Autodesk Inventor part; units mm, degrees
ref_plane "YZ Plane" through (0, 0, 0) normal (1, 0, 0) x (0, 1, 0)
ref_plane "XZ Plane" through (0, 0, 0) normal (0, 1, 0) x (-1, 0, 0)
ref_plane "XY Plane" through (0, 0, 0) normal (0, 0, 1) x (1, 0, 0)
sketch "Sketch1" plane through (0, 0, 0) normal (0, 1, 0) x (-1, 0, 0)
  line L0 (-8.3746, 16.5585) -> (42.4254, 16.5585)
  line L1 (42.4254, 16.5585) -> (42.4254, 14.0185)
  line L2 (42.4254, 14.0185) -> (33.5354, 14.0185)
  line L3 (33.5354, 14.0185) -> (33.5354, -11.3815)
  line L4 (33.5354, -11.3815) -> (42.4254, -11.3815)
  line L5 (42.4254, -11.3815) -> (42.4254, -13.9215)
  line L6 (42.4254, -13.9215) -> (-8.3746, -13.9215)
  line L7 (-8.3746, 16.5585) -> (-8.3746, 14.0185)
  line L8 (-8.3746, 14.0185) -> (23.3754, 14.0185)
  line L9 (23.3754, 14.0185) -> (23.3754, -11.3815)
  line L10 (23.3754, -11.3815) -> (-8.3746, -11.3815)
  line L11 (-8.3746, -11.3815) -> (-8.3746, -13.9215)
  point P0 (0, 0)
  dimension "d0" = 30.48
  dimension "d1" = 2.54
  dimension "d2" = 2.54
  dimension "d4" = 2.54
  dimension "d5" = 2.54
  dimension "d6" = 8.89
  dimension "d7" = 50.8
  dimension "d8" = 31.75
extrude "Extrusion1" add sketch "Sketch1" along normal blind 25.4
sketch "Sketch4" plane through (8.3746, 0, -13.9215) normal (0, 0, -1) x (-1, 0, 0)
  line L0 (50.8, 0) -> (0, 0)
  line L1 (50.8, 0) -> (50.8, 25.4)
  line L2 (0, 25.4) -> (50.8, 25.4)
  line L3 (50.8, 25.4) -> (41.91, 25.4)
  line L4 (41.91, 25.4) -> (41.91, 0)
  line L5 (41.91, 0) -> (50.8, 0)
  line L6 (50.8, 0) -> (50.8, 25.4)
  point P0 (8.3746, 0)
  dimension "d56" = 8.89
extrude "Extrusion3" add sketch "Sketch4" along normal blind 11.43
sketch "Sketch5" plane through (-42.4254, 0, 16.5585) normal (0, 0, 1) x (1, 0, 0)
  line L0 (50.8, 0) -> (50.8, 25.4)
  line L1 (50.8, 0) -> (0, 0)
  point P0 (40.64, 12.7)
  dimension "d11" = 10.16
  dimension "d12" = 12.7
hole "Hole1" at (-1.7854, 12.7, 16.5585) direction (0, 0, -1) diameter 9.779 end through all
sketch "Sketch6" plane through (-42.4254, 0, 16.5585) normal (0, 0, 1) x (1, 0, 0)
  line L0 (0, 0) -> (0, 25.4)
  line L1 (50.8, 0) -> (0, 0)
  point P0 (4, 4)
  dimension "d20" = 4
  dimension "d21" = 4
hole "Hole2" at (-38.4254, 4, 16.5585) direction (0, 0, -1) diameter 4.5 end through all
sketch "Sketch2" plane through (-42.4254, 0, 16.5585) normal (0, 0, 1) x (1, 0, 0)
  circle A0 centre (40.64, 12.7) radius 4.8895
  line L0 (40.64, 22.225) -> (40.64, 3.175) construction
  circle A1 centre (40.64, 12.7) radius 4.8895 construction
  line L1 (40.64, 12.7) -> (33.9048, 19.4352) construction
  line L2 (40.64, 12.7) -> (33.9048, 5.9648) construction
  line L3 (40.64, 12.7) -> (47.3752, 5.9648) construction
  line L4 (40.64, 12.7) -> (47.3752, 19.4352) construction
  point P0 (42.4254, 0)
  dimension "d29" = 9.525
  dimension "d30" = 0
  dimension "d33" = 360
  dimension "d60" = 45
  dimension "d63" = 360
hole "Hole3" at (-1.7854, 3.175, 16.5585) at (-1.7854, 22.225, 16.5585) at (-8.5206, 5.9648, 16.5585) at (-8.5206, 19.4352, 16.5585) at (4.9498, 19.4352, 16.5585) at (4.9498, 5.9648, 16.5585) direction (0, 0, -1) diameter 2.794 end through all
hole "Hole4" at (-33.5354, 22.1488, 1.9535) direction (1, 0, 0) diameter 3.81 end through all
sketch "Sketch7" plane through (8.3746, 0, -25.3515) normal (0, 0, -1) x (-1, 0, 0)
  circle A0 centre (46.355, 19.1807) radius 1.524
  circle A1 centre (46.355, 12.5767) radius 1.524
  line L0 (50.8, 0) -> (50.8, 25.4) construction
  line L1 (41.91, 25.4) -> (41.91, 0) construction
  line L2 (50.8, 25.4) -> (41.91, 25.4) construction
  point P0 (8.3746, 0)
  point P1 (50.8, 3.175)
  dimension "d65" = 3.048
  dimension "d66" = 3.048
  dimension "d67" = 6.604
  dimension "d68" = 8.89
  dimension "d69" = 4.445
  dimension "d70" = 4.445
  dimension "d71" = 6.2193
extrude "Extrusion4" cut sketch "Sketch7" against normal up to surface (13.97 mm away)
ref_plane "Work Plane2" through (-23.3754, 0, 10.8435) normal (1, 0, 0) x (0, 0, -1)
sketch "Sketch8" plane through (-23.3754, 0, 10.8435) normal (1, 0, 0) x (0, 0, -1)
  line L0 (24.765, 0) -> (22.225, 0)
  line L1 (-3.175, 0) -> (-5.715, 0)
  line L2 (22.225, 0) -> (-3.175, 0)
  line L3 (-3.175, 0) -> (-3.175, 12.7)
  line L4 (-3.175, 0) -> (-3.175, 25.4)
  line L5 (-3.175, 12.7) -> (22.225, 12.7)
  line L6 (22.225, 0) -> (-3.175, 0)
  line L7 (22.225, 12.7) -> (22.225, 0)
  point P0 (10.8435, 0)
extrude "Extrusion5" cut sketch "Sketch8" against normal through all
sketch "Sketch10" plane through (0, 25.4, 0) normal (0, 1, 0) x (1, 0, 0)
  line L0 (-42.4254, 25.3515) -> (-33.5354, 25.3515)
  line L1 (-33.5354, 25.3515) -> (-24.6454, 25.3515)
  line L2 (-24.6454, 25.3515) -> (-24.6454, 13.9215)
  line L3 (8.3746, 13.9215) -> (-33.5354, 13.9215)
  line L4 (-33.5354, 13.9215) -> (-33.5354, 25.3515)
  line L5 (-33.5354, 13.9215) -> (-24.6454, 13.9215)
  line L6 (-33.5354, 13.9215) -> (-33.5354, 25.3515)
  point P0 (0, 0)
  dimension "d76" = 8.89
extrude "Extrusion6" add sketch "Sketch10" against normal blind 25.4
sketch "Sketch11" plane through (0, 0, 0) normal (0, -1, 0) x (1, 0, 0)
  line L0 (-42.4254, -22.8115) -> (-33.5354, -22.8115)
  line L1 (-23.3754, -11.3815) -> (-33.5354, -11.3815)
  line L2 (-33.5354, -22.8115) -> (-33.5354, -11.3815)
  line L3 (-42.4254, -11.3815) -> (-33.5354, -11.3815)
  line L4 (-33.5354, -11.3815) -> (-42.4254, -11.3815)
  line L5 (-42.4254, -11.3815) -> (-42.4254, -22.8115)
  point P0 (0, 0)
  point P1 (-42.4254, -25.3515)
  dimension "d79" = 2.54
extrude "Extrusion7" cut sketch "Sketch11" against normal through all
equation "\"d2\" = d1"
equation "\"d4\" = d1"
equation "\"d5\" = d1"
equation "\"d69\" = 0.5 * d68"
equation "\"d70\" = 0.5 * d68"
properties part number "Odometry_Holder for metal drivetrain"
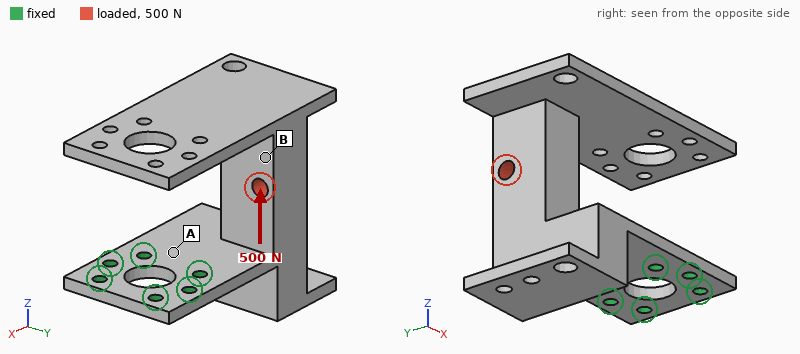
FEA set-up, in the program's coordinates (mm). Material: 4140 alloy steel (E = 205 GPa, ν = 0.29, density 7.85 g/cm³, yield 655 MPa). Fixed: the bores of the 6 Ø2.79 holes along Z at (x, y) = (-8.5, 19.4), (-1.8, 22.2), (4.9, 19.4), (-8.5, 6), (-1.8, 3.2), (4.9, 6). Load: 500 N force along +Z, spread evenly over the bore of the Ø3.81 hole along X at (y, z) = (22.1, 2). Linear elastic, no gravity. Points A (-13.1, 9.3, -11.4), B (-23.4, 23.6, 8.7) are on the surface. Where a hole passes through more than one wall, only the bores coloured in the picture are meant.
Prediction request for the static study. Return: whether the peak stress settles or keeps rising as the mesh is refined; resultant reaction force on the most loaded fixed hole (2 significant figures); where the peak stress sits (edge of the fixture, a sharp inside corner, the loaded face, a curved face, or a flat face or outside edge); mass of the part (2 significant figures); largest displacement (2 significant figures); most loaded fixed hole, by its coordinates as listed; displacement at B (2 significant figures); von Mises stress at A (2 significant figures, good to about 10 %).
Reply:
keeps rising
740 N
edge of the fixture
91 g
0.56 mm
(-8.5, 19.4)
0.32 mm
230 MPa
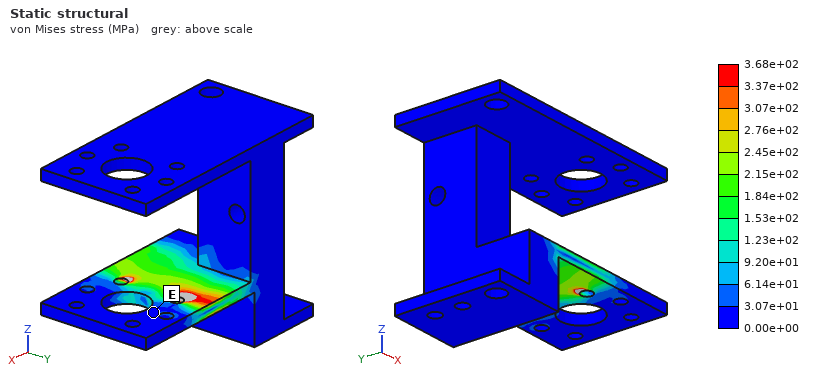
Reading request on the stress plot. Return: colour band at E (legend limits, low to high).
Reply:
0.00e+00 to 3.07e+01 MPa
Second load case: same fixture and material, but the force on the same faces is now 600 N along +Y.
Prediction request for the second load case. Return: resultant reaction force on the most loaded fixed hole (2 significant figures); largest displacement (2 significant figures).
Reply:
870 N
0.20 mm
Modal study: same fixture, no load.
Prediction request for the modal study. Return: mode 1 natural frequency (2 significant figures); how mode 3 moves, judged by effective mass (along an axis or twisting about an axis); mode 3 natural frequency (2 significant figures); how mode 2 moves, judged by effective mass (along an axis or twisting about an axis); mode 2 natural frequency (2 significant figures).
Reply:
530 Hz
along Z
1800 Hz
along Y
1100 Hz
